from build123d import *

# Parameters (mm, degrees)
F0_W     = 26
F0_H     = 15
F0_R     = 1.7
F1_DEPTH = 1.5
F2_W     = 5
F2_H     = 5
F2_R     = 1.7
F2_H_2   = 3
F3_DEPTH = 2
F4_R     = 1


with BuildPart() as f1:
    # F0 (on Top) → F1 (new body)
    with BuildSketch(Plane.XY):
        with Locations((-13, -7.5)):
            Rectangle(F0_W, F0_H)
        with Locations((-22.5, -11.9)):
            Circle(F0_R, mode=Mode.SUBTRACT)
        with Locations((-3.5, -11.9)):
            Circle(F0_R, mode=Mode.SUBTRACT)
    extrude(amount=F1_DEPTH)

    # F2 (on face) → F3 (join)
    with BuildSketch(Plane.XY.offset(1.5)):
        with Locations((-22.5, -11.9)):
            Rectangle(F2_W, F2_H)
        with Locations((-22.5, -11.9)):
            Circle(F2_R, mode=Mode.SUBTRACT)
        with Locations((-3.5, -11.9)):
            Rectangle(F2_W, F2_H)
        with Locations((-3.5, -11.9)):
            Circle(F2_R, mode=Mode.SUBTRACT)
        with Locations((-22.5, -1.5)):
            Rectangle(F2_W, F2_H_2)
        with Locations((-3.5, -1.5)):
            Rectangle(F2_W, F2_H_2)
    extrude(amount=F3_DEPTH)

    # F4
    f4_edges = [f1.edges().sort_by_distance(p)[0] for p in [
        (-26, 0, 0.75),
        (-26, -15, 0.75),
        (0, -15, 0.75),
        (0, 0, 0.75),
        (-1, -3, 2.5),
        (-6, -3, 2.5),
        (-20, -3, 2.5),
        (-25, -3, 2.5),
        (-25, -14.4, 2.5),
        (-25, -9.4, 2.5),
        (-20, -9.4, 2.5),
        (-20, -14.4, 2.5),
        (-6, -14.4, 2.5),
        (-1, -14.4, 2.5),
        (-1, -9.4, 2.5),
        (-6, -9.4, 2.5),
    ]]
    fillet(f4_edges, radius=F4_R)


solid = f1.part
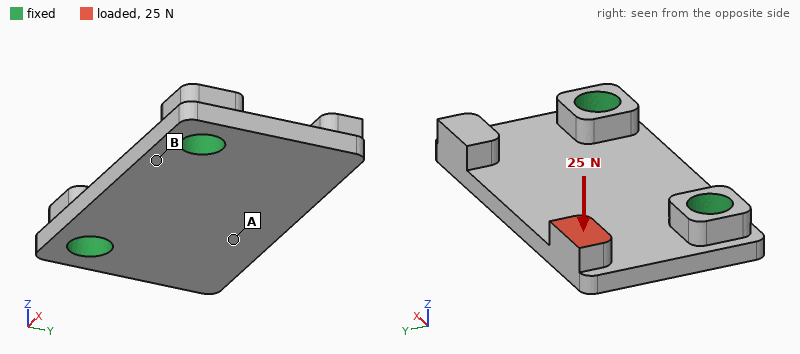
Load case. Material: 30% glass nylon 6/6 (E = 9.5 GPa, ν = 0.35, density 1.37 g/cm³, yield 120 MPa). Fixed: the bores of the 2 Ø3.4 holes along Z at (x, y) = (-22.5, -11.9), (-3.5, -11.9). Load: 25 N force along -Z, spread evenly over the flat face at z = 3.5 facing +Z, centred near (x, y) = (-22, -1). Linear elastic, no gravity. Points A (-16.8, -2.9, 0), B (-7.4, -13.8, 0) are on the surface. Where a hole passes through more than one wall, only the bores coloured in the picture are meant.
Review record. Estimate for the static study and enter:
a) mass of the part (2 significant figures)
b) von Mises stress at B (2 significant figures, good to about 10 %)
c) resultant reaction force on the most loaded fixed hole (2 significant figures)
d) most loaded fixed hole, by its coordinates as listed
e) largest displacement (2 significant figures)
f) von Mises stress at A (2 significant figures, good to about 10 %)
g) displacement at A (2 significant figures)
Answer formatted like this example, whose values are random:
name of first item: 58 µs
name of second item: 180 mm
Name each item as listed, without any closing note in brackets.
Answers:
mass of the part: 0.92 g
von Mises stress at B: 4.7 MPa
resultant reaction force on the most loaded fixed hole: 25 N
most loaded fixed hole, by its coordinates as listed: (-22.5, -11.9)
largest displacement: 0.23 mm
von Mises stress at A: 17 MPa
displacement at A: 0.098 mm
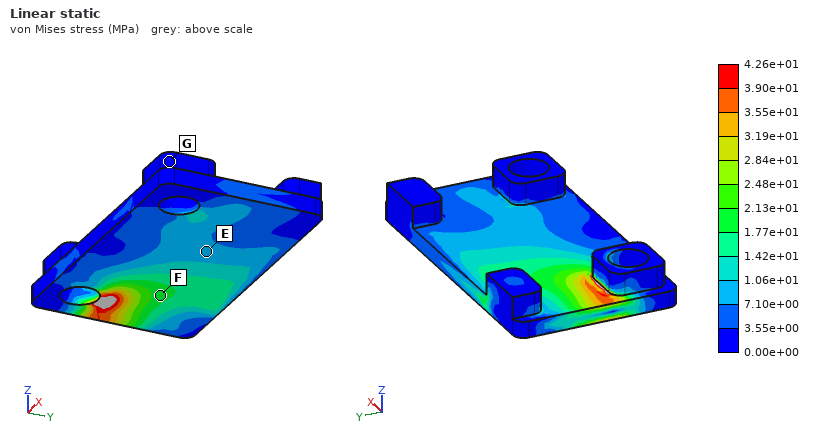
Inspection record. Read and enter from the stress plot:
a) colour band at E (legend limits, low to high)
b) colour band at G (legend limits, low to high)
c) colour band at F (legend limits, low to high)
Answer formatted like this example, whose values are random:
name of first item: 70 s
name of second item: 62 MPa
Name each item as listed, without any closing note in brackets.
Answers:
colour band at E: 7.10e+00 to 1.06e+01 MPa
colour band at G: 0.00e+00 to 3.55e+00 MPa
colour band at F: 1.77e+01 to 2.13e+01 MPa
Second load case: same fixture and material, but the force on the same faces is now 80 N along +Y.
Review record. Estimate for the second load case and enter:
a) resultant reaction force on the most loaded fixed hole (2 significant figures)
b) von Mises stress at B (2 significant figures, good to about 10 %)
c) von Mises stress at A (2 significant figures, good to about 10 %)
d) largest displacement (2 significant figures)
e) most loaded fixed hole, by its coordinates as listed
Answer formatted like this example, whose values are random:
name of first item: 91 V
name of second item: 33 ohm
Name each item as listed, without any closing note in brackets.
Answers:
resultant reaction force on the most loaded fixed hole: 79 N
von Mises stress at B: 5.8 MPa
von Mises stress at A: 35 MPa
largest displacement: 0.35 mm
most loaded fixed hole, by its coordinates as listed: (-22.5, -11.9)
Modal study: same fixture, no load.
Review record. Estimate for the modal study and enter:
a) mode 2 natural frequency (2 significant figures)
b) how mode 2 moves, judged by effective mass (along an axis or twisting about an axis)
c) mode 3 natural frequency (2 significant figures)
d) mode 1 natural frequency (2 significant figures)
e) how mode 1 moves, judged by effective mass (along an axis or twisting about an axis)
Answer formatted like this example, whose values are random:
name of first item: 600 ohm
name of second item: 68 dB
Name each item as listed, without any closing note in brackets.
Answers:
mode 2 natural frequency: 6500 Hz
how mode 2 moves, judged by effective mass: twisting about Y
mode 3 natural frequency: 10 kHz
mode 1 natural frequency: 4500 Hz
how mode 1 moves, judged by effective mass: along Z
